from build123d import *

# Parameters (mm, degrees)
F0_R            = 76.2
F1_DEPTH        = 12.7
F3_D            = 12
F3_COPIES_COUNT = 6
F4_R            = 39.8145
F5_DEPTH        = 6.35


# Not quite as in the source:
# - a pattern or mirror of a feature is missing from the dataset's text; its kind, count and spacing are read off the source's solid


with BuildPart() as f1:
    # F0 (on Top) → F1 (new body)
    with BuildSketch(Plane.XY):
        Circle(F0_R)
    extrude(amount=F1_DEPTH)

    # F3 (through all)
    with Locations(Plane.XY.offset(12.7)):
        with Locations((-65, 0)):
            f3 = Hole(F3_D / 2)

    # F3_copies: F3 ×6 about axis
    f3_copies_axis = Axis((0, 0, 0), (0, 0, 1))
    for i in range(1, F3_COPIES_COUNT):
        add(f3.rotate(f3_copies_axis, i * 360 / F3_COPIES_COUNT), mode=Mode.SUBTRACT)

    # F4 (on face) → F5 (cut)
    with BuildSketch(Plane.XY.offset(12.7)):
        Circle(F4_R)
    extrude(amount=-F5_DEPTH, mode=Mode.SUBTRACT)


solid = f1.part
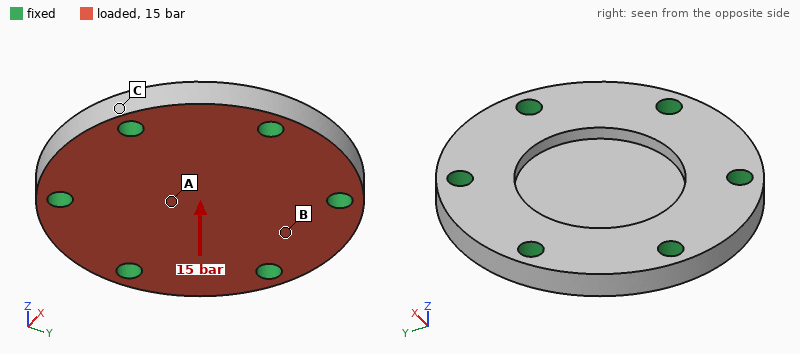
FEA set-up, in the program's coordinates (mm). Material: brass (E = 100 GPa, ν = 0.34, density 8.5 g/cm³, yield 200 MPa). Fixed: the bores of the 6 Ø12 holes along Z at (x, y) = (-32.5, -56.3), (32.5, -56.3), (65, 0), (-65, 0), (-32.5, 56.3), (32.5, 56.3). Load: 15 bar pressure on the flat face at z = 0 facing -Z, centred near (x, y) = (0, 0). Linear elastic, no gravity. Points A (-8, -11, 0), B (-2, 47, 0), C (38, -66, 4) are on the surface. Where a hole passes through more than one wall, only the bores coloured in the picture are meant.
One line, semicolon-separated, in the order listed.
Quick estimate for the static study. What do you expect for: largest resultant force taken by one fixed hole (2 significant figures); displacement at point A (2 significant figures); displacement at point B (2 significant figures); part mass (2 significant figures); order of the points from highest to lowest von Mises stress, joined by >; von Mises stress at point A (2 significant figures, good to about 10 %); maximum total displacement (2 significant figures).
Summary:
4.6 kN; 55 µm; 12 µm; 1.6 kg; A > B > C; 39 MPa; 63 µm
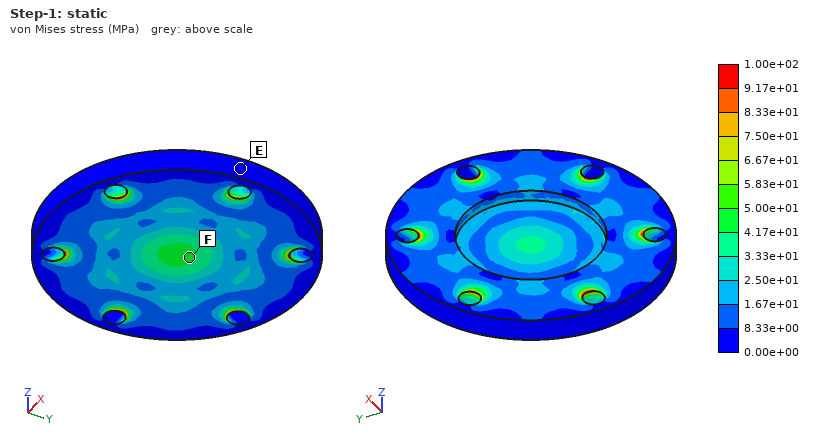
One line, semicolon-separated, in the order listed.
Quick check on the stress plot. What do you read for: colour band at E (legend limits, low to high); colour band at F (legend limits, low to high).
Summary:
0.00e+00 to 8.33e+00 MPa; 4.17e+01 to 5.00e+01 MPa
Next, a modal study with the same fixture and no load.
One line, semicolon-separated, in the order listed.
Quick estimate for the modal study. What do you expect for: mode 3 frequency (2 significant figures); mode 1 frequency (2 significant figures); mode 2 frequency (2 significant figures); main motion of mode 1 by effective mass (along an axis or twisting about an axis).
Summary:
7100 Hz; 4200 Hz; 7100 Hz; along Z
